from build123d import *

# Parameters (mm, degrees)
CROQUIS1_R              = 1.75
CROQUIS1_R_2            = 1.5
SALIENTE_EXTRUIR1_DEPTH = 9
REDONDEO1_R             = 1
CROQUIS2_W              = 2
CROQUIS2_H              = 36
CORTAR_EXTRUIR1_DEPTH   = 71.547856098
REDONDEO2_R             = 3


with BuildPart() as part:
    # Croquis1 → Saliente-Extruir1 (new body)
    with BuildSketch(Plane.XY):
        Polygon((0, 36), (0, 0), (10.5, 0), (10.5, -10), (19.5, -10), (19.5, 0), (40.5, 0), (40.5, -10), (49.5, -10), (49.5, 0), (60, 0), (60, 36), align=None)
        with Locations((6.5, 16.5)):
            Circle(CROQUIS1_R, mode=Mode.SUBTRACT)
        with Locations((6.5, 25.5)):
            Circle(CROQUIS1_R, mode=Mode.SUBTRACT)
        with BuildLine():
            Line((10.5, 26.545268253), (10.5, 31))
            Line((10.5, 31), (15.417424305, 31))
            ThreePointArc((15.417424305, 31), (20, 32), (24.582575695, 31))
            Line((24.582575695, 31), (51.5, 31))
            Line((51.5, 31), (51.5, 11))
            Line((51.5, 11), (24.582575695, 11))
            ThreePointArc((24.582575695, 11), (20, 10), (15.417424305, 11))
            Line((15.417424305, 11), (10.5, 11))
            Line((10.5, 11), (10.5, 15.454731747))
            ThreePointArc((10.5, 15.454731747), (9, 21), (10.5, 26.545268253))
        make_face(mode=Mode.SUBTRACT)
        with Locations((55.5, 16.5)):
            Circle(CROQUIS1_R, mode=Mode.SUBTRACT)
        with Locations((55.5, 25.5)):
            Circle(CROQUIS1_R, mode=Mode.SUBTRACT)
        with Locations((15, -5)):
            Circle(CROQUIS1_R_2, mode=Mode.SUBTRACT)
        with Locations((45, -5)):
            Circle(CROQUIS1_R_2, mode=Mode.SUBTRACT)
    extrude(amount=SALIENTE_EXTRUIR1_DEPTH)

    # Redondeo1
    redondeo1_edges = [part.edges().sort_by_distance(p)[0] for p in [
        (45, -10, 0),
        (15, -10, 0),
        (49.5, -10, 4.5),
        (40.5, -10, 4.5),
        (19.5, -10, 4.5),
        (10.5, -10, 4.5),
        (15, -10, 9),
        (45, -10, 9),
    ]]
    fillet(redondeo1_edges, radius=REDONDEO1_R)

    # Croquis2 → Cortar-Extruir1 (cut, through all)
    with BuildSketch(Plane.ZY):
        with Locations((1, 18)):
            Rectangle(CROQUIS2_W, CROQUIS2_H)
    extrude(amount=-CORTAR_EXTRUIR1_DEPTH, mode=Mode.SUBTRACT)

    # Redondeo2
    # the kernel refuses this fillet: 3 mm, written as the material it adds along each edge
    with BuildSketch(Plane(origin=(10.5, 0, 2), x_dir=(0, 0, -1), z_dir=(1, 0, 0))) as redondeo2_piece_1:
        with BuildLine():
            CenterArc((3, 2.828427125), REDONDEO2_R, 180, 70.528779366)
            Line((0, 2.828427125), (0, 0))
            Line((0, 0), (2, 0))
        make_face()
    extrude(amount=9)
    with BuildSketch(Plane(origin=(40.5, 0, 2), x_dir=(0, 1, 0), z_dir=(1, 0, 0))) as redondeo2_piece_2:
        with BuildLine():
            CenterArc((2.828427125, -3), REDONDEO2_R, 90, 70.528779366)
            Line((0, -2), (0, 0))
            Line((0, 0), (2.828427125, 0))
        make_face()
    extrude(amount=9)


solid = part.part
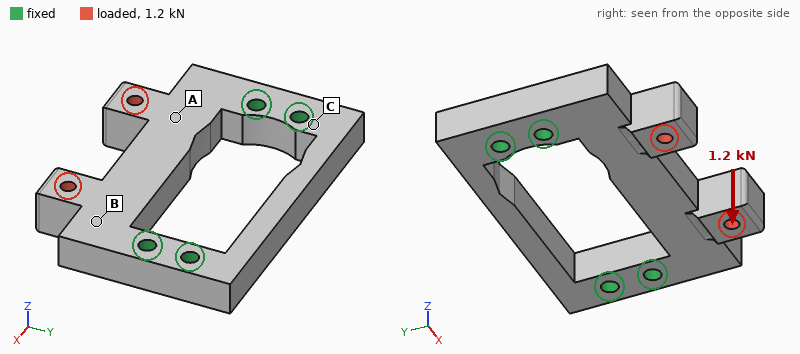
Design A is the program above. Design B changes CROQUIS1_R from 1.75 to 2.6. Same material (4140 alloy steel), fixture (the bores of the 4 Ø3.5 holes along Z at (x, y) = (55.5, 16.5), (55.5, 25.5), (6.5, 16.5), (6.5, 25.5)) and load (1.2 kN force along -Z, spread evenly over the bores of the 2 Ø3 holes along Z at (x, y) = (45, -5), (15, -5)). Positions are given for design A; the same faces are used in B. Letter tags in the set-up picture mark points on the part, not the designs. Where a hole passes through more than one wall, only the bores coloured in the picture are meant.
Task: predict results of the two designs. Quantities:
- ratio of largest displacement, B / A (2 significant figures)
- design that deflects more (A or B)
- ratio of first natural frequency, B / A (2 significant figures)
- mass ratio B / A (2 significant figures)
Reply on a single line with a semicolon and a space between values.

0.88; A; 1.1; 0.97
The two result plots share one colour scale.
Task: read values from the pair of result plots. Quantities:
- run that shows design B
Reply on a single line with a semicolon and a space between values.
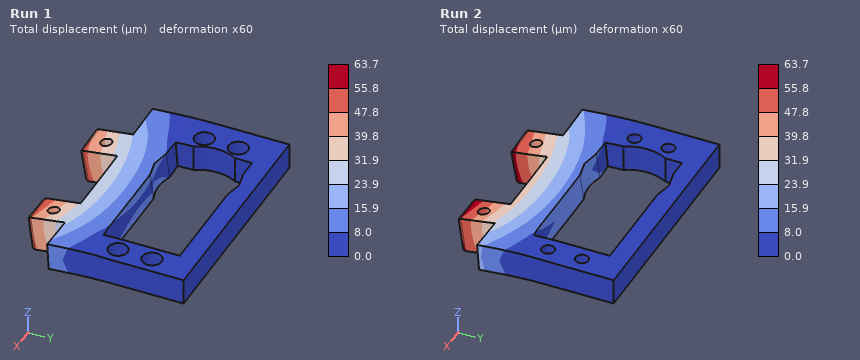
Run 1
